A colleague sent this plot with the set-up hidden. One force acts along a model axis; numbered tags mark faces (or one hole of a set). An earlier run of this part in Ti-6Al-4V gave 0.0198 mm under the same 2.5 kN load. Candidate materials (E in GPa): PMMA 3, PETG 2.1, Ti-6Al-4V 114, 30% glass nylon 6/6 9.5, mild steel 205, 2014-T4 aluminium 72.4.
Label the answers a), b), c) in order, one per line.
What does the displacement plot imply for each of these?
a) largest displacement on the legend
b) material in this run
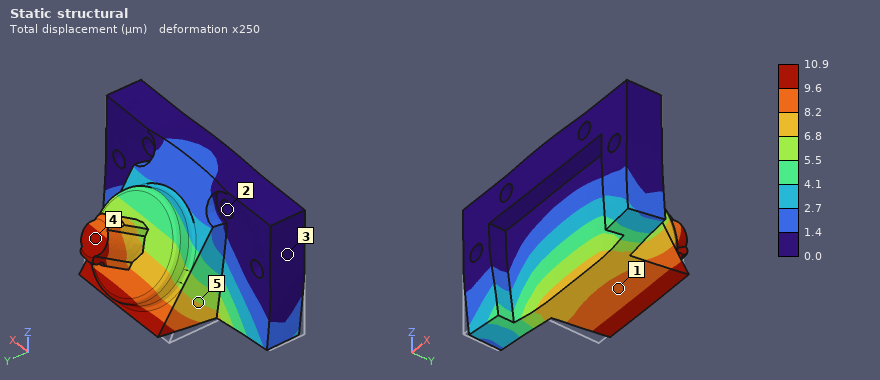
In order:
a) 10.9 µm
b) mild steel
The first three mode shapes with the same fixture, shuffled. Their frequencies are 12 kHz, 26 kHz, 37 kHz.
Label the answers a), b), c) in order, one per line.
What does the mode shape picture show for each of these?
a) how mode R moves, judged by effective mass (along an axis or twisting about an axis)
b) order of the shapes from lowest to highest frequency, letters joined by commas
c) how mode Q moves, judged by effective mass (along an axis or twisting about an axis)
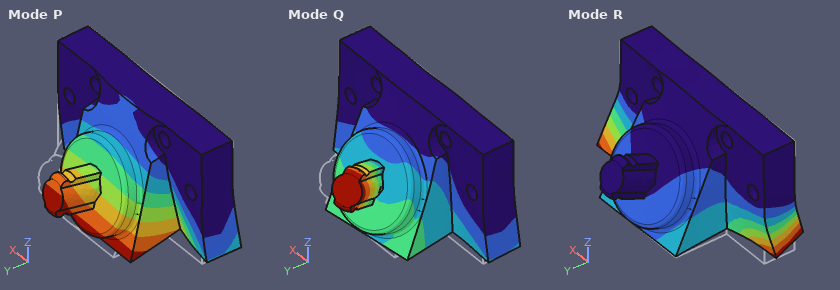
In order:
a) along X
b) P, Q, R
c) along X
